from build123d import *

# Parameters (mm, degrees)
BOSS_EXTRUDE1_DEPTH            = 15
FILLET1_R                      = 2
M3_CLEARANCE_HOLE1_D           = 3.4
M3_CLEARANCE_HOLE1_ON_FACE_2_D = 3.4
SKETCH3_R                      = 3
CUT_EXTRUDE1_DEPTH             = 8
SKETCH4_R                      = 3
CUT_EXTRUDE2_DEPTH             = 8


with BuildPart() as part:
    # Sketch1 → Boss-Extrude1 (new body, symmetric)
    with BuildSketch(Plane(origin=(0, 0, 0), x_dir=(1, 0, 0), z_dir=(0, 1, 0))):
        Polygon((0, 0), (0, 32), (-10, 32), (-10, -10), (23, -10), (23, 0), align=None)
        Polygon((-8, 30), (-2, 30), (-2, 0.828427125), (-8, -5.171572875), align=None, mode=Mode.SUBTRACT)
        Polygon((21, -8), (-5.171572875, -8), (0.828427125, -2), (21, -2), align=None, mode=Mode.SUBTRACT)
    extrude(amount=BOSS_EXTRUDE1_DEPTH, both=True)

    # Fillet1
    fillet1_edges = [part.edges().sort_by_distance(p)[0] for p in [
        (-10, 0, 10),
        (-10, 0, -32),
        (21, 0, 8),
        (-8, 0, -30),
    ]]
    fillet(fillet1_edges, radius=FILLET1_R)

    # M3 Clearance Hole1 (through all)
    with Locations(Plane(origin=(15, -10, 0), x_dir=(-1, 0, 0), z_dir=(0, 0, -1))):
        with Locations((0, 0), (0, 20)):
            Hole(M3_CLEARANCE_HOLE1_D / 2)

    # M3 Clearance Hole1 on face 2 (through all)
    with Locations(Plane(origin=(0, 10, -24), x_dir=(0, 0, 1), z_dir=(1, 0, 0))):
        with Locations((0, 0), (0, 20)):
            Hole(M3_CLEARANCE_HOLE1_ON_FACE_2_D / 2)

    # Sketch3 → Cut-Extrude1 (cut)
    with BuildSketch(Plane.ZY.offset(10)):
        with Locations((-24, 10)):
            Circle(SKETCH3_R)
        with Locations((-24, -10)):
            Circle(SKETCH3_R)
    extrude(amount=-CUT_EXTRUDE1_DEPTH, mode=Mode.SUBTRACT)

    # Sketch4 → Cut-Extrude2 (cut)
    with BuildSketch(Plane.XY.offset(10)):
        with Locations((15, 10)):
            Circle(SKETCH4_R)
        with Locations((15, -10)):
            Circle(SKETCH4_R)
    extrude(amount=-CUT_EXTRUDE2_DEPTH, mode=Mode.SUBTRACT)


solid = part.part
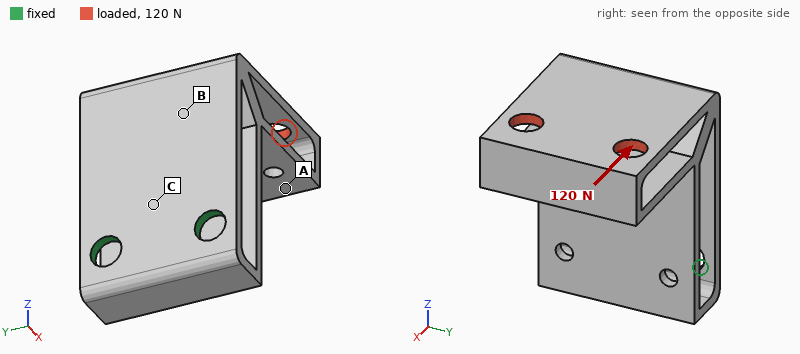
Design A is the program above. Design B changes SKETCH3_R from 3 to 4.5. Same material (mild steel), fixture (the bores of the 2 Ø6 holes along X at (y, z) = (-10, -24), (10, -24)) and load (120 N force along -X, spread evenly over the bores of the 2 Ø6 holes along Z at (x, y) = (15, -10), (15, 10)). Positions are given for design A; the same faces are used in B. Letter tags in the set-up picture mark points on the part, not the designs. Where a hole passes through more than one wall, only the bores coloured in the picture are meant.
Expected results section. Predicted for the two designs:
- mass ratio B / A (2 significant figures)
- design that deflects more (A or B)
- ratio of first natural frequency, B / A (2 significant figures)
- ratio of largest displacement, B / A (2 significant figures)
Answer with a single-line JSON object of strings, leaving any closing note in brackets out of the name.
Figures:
{"mass ratio B / A": "0.98", "design that deflects more": "A", "ratio of first natural frequency, B / A": "1.2", "ratio of largest displacement, B / A": "0.73"}
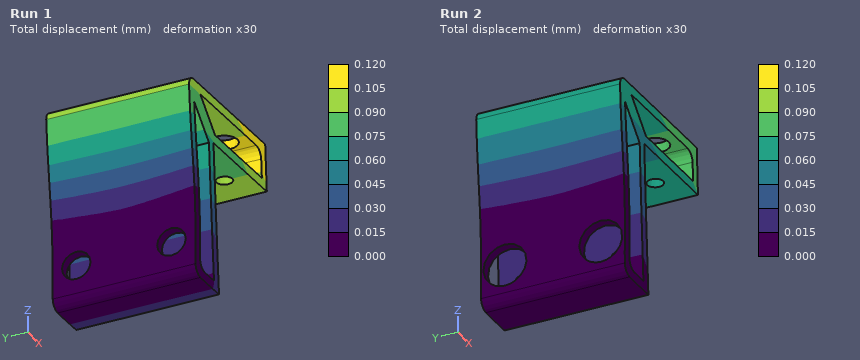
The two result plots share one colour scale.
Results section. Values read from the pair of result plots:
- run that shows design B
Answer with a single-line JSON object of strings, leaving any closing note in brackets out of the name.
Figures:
{"run that shows design B": "Run 2"}
